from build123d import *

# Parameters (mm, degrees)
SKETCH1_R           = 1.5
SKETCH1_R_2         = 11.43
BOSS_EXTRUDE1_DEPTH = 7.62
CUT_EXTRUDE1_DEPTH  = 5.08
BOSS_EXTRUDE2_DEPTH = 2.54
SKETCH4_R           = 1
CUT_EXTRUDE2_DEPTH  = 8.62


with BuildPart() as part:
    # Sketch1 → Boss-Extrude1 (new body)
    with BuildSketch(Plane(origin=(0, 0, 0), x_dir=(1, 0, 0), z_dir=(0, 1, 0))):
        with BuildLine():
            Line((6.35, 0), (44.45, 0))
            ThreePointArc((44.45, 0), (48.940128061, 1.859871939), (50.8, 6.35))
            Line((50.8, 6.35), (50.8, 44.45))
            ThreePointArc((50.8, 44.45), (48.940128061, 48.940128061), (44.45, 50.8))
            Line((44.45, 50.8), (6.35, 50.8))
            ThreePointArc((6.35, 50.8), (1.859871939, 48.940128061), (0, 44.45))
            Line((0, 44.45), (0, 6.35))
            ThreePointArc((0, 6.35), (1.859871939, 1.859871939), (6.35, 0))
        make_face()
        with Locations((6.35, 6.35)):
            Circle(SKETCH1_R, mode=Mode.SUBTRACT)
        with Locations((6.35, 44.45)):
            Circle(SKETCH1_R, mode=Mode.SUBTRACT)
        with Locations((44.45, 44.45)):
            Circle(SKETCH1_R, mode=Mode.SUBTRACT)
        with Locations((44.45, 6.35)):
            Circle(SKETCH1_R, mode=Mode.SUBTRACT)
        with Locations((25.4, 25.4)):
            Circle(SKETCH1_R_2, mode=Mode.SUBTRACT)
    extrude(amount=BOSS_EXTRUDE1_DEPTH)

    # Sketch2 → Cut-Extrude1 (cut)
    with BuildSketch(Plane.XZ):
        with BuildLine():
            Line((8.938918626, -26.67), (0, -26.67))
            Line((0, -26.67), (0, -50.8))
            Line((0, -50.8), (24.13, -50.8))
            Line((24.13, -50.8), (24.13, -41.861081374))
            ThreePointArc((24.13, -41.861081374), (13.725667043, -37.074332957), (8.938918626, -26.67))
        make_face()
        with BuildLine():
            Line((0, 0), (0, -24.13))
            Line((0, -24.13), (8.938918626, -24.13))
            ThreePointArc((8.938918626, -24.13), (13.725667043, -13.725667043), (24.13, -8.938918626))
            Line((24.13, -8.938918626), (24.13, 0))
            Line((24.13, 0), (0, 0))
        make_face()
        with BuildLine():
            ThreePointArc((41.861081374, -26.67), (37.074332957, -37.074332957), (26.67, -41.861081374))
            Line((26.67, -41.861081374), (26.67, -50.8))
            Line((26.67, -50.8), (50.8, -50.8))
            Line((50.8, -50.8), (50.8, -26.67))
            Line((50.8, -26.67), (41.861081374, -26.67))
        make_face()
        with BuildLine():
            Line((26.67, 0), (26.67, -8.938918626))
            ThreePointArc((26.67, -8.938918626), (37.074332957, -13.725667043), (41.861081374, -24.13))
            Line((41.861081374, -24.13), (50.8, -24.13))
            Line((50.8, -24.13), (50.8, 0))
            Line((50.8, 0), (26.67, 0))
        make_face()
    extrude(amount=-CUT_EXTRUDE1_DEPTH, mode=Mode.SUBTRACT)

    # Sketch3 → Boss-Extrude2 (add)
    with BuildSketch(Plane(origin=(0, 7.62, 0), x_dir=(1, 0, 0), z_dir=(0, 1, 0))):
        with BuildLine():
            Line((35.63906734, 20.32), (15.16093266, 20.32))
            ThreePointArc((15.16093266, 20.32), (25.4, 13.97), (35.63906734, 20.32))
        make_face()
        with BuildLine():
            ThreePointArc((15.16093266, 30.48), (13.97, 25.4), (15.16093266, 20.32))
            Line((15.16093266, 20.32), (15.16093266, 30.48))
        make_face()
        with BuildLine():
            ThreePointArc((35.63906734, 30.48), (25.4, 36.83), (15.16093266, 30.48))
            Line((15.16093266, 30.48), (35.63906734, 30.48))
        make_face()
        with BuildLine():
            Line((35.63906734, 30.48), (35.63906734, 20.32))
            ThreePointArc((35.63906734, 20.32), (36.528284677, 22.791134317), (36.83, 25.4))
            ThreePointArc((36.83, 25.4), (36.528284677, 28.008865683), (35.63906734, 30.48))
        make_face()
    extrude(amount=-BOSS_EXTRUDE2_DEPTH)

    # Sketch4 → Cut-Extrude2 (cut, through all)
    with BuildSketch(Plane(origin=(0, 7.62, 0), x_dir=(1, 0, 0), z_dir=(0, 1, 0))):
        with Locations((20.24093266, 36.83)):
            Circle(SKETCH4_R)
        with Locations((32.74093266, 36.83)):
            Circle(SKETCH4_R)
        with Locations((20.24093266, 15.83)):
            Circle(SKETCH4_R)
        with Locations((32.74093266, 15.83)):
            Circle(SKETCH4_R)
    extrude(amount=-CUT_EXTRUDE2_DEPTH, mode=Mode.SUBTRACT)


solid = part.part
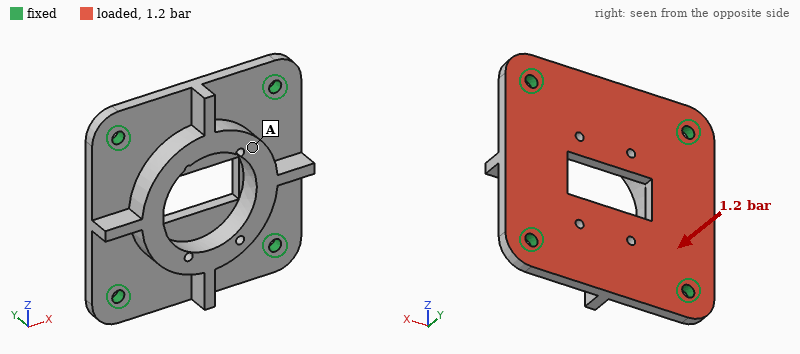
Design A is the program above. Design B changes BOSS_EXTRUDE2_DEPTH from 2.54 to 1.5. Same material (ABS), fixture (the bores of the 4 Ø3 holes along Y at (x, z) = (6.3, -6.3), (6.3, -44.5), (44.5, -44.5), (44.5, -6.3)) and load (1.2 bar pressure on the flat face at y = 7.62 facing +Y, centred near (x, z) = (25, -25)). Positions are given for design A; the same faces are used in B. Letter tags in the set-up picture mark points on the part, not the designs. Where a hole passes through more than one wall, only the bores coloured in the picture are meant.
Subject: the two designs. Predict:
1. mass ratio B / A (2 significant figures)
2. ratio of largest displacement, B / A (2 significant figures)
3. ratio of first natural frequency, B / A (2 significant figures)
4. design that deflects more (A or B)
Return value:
0.98
1.1
1.0
B
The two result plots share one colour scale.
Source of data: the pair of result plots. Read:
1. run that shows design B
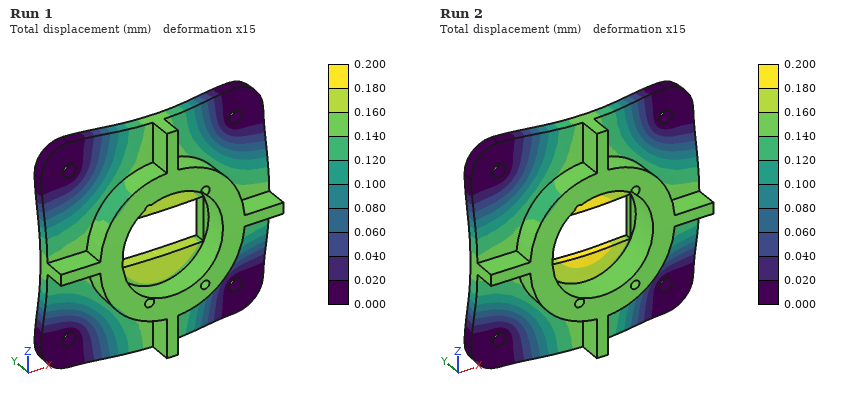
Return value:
Run 2
